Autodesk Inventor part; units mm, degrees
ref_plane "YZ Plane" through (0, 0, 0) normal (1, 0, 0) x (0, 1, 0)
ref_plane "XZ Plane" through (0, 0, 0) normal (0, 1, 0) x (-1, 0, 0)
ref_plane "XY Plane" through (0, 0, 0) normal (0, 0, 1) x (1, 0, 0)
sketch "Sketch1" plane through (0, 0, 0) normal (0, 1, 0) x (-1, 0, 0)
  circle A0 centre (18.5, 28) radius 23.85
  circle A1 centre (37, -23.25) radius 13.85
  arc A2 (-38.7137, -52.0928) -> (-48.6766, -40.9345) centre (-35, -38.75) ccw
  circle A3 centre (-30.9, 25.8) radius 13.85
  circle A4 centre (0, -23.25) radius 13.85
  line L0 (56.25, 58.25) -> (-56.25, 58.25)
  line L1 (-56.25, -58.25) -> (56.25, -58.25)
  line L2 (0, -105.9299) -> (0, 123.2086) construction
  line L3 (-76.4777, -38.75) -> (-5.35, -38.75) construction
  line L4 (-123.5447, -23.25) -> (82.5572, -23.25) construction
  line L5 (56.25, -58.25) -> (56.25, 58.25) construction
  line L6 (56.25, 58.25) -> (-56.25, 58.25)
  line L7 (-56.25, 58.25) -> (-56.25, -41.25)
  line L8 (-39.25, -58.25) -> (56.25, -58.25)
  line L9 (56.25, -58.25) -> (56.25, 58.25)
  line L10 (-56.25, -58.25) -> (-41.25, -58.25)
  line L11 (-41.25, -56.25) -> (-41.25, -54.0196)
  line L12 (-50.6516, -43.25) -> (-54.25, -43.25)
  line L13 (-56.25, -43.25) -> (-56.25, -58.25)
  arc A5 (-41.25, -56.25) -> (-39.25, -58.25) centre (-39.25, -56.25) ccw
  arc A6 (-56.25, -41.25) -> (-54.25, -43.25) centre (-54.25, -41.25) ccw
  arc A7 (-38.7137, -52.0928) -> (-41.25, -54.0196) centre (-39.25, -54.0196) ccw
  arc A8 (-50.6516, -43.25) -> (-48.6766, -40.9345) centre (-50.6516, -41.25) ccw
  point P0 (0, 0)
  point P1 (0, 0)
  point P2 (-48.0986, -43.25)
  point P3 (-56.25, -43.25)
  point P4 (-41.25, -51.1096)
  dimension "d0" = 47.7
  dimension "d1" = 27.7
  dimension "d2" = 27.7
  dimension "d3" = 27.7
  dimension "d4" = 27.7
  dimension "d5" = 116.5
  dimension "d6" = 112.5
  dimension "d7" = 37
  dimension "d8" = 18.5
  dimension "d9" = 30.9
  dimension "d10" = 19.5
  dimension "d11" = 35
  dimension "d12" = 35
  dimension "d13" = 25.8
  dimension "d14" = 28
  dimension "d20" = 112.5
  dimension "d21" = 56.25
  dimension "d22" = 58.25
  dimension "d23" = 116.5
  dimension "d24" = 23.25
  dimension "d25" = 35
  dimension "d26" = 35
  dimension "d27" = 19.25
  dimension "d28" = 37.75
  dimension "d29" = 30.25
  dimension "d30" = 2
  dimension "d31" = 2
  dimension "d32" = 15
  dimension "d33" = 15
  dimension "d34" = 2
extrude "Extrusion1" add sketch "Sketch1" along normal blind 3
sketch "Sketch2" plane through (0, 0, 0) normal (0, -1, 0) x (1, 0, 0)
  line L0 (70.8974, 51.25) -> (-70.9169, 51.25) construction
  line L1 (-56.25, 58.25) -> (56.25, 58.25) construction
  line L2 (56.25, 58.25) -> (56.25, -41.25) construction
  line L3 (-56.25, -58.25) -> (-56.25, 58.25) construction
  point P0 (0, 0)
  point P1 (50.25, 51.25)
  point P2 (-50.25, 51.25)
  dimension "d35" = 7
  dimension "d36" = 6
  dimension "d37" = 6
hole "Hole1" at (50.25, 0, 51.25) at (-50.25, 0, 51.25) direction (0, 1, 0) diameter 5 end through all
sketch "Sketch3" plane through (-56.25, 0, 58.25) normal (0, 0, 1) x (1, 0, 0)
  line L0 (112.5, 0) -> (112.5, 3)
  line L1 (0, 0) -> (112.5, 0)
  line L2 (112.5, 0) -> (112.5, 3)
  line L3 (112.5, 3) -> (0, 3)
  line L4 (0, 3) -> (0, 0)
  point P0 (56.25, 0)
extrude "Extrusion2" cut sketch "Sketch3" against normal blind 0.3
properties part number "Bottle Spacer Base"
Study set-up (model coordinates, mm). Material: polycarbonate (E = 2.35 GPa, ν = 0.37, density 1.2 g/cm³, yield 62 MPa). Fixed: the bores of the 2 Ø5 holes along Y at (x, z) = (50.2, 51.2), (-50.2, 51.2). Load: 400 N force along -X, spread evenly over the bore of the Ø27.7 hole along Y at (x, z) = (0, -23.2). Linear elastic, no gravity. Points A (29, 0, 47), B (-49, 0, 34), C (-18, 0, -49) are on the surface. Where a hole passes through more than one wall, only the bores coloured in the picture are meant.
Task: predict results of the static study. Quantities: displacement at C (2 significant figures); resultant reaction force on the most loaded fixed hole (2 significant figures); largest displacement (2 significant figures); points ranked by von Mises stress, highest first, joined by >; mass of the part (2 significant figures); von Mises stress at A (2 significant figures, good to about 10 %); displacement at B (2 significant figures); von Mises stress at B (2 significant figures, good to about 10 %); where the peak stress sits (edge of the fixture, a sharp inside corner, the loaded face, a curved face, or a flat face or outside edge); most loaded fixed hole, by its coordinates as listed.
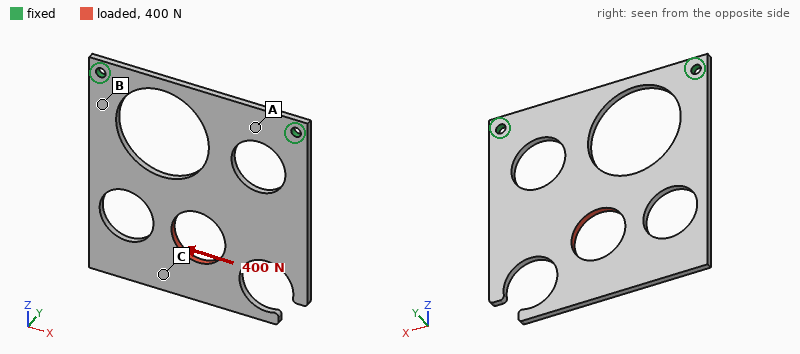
0.80 mm
370 N
0.85 mm
B > A > C
31 g
5.9 MPa
0.21 mm
10.0 MPa
edge of the fixture
(50.2, 51.2)
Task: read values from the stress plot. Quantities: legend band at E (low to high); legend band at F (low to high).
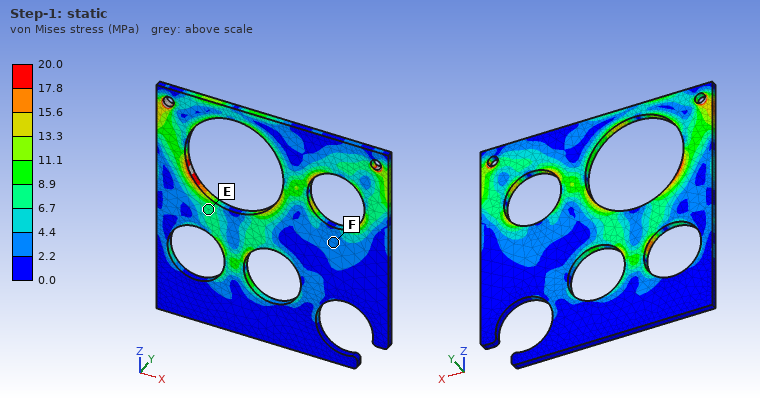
6.7 to 8.9 MPa
2.2 to 4.4 MPa
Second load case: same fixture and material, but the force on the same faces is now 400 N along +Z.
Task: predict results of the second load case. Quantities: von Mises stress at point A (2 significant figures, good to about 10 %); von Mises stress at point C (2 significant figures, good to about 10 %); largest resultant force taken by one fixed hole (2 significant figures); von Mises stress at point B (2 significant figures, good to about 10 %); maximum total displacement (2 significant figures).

3.0 MPa
1.1 MPa
210 N
5.7 MPa
0.28 mm
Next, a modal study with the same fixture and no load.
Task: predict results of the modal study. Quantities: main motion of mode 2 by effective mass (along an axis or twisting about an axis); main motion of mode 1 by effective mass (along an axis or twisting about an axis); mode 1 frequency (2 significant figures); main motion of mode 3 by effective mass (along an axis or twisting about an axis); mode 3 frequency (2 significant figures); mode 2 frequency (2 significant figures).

twisting about Z
along Y
42 Hz
along Y
260 Hz
130 Hz
